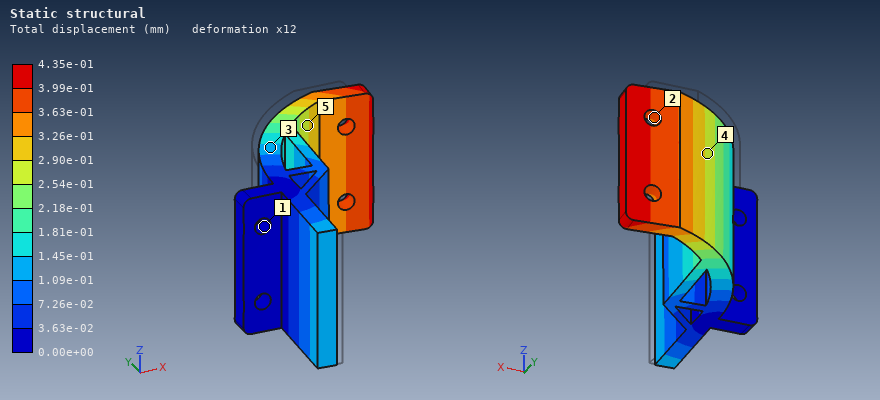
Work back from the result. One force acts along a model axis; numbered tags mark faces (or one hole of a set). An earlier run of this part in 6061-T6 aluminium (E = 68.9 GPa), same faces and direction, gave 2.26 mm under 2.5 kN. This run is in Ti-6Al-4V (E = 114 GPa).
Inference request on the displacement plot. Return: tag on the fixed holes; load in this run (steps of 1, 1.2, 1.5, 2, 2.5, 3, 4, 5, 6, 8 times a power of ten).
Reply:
1
800 N
